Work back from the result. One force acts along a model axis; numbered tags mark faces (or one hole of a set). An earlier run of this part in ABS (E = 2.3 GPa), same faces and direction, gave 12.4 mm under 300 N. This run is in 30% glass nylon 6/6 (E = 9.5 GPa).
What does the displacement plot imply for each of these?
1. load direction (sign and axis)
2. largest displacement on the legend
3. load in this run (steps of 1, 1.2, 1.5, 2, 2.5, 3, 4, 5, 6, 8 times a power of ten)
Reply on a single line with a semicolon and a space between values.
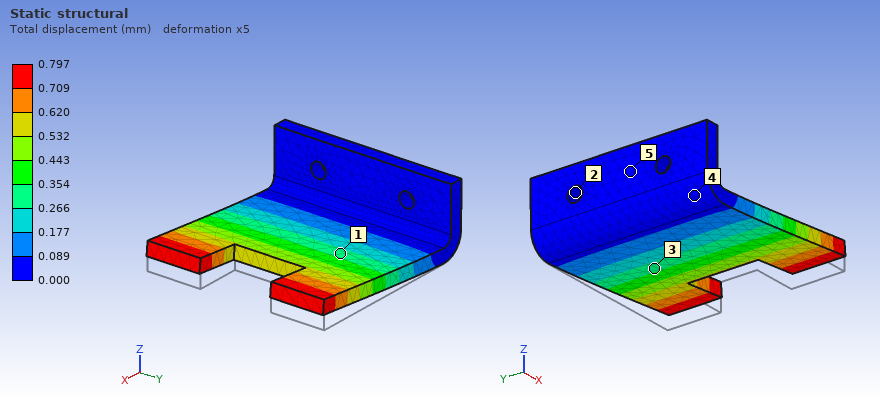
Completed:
+Z; 0.797 mm; 80 N
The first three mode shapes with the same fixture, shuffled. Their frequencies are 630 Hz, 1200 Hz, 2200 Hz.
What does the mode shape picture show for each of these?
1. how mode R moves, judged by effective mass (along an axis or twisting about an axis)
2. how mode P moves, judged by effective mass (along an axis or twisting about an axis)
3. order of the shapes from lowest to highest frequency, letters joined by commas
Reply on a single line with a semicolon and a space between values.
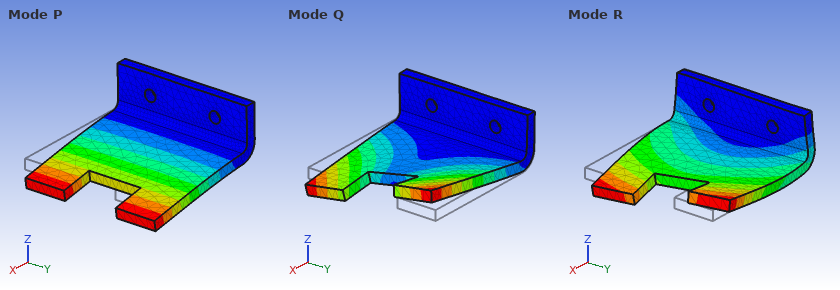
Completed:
along Y; along Z; P, Q, R
